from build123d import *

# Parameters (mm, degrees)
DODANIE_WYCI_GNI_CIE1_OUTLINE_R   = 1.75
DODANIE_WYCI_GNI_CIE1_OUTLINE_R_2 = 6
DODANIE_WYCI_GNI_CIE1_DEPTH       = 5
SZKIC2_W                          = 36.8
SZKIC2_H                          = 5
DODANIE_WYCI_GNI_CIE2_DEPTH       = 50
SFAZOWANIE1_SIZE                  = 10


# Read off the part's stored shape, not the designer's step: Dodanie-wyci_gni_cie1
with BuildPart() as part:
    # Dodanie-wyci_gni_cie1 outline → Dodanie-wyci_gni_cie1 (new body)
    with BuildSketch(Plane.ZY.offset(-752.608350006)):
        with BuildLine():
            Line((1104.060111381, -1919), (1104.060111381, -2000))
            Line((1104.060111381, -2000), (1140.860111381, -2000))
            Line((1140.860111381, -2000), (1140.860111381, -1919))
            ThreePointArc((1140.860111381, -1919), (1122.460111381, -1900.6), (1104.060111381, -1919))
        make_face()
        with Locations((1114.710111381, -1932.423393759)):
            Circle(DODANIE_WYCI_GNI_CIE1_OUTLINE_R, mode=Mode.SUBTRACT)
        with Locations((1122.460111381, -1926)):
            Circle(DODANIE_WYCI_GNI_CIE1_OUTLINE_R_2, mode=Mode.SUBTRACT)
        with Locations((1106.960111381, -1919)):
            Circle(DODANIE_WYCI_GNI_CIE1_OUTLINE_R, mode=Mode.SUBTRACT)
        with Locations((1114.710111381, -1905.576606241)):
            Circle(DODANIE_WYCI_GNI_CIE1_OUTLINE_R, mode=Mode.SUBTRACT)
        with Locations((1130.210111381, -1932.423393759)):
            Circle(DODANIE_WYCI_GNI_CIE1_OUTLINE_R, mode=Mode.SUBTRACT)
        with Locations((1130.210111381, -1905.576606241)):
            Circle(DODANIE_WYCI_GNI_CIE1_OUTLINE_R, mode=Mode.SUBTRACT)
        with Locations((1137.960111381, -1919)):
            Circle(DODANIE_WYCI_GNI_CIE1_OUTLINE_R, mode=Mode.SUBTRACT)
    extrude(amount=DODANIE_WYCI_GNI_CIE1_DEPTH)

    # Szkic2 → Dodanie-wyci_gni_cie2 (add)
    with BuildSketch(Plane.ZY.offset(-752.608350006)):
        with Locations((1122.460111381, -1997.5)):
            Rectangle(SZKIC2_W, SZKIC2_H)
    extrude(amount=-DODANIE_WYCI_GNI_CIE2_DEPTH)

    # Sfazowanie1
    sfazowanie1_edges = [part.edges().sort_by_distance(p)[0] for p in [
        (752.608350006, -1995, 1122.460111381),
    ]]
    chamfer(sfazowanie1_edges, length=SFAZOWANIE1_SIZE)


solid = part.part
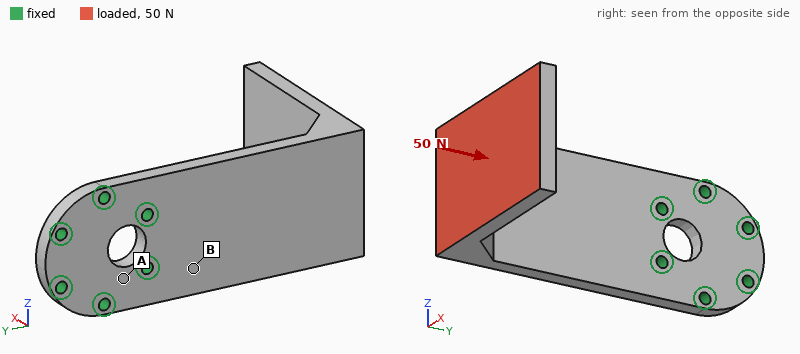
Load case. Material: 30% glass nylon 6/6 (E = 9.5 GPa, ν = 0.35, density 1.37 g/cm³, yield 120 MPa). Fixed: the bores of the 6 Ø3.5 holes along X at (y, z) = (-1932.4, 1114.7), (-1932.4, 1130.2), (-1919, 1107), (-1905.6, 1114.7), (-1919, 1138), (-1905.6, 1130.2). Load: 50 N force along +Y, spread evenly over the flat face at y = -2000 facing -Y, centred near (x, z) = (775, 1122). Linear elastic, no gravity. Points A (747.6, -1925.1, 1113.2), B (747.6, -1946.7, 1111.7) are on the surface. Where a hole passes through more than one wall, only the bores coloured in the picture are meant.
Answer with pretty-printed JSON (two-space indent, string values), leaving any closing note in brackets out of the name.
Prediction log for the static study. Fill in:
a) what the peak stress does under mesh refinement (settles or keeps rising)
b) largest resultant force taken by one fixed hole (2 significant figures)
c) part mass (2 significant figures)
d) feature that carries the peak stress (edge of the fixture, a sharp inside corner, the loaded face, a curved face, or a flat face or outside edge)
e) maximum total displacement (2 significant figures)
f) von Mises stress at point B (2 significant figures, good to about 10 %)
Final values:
{
  "what the peak stress does under mesh refinement": "keeps rising",
  "largest resultant force taken by one fixed hole": "25 N",
  "part mass": "38 g",
  "feature that carries the peak stress": "edge of the fixture",
  "maximum total displacement": "1.3 mm",
  "von Mises stress at point B": "7.6 MPa"
}
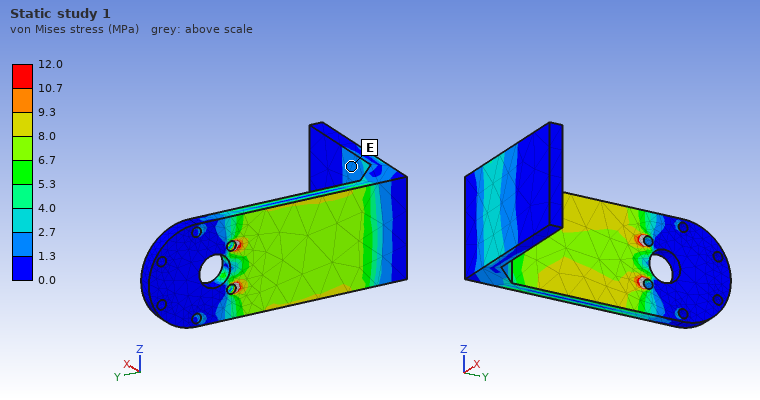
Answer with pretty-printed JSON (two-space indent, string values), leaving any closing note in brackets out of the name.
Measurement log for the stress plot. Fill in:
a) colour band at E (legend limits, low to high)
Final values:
{
  "colour band at E": "1.3 to 2.7 MPa"
}
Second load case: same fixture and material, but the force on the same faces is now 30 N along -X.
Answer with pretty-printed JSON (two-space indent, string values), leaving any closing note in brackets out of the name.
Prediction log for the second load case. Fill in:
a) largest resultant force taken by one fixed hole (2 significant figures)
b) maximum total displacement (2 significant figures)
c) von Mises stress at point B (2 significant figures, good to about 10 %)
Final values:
{
  "largest resultant force taken by one fixed hole": "37 N",
  "maximum total displacement": "1.3 mm",
  "von Mises stress at point B": "9.9 MPa"
}
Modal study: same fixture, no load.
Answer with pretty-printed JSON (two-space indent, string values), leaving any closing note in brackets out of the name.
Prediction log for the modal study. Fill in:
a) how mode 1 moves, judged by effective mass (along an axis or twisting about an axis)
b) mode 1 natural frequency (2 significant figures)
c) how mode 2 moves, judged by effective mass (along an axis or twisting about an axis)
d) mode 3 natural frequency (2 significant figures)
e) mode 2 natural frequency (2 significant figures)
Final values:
{
  "how mode 1 moves, judged by effective mass": "along X",
  "mode 1 natural frequency": "200 Hz",
  "how mode 2 moves, judged by effective mass": "along Z",
  "mode 3 natural frequency": "780 Hz",
  "mode 2 natural frequency": "440 Hz"
}
